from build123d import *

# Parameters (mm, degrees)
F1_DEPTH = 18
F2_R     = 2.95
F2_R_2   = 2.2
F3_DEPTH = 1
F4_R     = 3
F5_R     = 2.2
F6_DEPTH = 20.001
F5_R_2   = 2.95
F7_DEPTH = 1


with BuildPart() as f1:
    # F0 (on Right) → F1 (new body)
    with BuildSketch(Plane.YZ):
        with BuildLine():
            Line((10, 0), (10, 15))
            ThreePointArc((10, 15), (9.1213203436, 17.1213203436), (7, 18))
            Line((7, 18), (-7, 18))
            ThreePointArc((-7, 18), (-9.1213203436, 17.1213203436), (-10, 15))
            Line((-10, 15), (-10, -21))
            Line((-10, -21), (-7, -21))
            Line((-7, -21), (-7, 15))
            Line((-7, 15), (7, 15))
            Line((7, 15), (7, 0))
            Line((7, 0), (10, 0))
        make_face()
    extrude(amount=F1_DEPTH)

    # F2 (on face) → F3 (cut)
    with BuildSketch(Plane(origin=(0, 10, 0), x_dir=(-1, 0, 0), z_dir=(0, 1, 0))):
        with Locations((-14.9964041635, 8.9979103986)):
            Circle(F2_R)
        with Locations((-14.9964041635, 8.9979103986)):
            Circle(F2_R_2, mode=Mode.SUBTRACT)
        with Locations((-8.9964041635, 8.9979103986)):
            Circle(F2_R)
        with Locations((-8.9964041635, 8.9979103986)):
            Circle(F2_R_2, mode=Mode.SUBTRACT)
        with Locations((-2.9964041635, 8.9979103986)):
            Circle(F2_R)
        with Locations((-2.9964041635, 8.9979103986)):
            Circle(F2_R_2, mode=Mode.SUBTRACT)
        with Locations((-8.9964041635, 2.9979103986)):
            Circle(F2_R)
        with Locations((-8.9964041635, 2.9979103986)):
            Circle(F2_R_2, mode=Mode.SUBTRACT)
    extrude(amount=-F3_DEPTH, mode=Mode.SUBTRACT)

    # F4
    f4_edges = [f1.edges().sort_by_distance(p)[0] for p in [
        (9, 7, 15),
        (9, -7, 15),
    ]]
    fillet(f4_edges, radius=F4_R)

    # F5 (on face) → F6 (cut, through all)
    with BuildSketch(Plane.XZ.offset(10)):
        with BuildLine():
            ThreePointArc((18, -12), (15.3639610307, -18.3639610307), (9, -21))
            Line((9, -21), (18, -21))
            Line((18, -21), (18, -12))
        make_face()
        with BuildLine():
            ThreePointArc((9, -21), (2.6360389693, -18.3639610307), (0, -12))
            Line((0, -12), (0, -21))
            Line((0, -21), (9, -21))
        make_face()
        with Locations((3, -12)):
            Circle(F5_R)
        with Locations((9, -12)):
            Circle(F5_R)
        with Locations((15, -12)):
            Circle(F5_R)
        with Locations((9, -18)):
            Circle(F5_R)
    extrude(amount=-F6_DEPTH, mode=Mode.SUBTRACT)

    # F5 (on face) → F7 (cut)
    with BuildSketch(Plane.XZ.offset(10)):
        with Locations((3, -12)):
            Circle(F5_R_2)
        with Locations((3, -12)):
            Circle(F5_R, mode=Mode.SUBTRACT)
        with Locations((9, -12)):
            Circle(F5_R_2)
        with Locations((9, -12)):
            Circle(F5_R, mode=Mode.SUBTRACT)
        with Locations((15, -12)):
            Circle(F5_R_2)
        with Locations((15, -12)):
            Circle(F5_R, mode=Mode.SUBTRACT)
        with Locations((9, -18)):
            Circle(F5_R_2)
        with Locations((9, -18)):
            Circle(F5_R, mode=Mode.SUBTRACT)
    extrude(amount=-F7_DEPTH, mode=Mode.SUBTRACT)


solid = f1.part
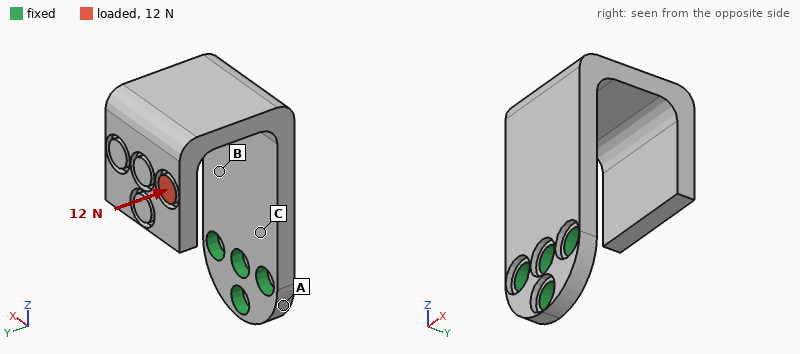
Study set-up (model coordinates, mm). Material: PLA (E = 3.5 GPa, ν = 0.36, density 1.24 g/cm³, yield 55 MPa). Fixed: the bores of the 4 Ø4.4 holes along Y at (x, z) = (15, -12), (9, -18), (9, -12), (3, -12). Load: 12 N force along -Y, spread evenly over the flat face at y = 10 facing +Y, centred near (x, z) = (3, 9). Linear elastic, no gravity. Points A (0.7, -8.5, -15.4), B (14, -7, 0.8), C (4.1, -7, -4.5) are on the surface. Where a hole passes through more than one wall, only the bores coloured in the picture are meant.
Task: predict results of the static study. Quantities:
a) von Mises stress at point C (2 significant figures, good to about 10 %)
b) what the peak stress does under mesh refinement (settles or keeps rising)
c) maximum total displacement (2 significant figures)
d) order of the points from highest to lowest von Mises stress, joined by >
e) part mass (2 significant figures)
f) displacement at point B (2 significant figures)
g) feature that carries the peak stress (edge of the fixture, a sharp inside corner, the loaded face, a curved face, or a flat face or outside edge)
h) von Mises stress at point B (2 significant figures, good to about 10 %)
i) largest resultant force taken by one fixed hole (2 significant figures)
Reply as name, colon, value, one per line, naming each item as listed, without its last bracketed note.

von Mises stress at point C: 6.2 MPa
what the peak stress does under mesh refinement: keeps rising
maximum total displacement: 0.54 mm
order of the points from highest to lowest von Mises stress, joined by >: C > B > A
part mass: 4.3 g
displacement at point B: 0.098 mm
feature that carries the peak stress: edge of the fixture
von Mises stress at point B: 4.0 MPa
largest resultant force taken by one fixed hole: 8.1 N
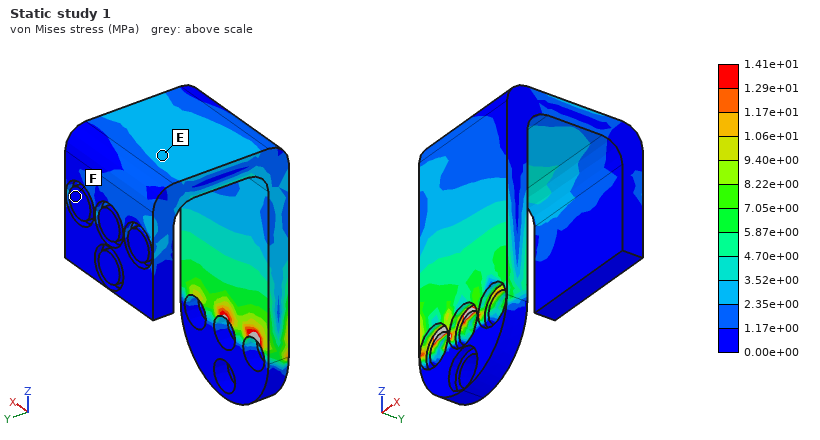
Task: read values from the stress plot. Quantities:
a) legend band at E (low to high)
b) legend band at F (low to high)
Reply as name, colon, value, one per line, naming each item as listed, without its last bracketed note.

legend band at E: 2.35e+00 to 3.52e+00 MPa
legend band at F: 0.00e+00 to 1.17e+00 MPa
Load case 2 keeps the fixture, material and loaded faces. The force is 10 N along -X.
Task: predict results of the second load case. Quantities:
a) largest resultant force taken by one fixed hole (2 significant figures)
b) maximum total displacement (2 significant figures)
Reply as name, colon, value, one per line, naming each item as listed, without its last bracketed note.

largest resultant force taken by one fixed hole: 19 N
maximum total displacement: 0.53 mm
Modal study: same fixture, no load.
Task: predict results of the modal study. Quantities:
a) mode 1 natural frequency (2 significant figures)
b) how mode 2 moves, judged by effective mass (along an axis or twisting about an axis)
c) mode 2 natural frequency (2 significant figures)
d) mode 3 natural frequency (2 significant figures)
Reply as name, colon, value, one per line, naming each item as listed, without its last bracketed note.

mode 1 natural frequency: 390 Hz
how mode 2 moves, judged by effective mass: along X
mode 2 natural frequency: 640 Hz
mode 3 natural frequency: 900 Hz
